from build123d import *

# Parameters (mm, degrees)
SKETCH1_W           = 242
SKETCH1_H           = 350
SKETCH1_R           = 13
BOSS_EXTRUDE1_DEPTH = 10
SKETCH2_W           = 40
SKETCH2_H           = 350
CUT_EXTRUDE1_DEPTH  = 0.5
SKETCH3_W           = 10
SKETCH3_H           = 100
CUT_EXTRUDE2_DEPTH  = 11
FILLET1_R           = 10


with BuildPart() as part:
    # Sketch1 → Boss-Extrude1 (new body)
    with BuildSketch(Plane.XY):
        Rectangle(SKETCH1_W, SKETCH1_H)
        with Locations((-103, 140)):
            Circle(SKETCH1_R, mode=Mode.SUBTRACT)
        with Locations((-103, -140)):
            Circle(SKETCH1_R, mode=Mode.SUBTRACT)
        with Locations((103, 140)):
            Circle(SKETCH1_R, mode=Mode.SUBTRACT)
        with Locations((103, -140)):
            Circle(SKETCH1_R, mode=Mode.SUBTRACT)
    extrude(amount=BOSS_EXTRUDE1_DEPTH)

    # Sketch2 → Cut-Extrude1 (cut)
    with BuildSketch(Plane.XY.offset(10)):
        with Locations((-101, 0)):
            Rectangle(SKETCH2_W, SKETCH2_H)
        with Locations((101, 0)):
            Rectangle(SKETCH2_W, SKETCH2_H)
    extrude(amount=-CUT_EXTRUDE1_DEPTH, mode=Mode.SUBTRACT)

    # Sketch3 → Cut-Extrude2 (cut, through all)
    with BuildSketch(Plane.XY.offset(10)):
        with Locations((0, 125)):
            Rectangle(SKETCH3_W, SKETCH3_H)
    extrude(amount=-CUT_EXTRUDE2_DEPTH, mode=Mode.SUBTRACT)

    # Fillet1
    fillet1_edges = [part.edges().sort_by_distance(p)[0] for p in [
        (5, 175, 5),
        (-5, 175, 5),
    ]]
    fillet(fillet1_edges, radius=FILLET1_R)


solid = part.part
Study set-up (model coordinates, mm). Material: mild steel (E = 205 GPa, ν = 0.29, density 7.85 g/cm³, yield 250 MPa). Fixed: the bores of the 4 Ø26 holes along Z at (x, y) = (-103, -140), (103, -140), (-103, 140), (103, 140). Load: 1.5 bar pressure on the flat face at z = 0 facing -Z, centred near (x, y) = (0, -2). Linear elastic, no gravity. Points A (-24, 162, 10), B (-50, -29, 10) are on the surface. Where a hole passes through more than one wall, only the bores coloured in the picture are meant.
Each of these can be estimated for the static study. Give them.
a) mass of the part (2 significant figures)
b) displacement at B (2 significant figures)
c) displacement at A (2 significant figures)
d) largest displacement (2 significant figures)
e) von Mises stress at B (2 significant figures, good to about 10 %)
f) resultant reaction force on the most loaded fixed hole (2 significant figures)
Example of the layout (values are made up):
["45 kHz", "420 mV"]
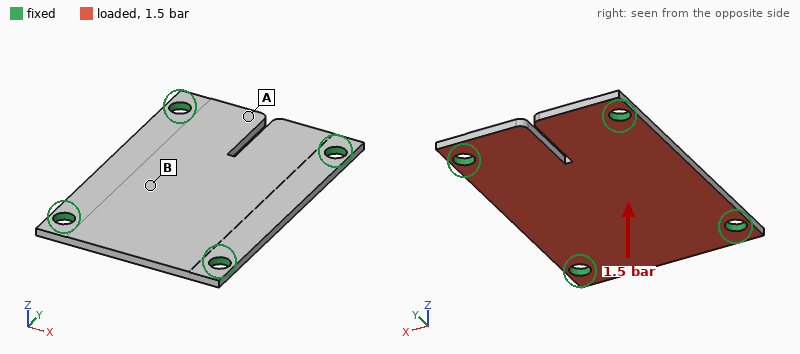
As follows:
["6.3 kg", "0.17 mm", "0.046 mm", "0.20 mm", "26 MPa", "3.1 kN"]
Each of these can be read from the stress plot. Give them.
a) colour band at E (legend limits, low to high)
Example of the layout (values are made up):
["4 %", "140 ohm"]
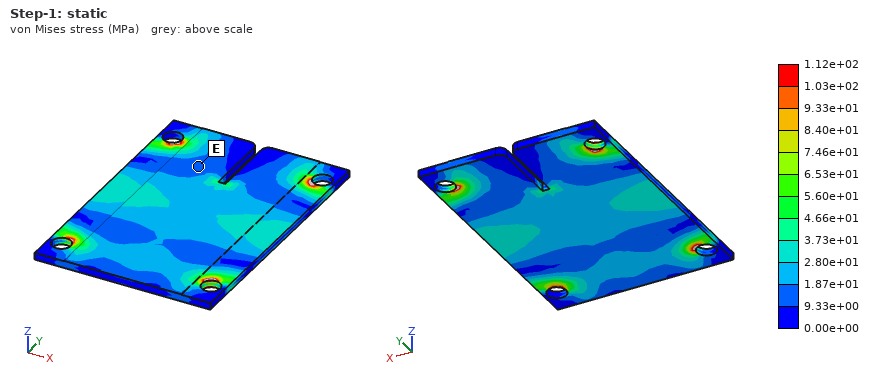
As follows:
["9.33e+00 to 1.87e+01 MPa"]
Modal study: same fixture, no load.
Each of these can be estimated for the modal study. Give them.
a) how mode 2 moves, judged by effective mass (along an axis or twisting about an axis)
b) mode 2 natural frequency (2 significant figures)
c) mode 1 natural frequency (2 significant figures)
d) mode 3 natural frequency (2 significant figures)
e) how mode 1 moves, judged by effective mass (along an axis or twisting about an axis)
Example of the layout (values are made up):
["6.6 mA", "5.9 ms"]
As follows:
["twisting about Y", "890 Hz", "590 Hz", "1100 Hz", "along Z"]
